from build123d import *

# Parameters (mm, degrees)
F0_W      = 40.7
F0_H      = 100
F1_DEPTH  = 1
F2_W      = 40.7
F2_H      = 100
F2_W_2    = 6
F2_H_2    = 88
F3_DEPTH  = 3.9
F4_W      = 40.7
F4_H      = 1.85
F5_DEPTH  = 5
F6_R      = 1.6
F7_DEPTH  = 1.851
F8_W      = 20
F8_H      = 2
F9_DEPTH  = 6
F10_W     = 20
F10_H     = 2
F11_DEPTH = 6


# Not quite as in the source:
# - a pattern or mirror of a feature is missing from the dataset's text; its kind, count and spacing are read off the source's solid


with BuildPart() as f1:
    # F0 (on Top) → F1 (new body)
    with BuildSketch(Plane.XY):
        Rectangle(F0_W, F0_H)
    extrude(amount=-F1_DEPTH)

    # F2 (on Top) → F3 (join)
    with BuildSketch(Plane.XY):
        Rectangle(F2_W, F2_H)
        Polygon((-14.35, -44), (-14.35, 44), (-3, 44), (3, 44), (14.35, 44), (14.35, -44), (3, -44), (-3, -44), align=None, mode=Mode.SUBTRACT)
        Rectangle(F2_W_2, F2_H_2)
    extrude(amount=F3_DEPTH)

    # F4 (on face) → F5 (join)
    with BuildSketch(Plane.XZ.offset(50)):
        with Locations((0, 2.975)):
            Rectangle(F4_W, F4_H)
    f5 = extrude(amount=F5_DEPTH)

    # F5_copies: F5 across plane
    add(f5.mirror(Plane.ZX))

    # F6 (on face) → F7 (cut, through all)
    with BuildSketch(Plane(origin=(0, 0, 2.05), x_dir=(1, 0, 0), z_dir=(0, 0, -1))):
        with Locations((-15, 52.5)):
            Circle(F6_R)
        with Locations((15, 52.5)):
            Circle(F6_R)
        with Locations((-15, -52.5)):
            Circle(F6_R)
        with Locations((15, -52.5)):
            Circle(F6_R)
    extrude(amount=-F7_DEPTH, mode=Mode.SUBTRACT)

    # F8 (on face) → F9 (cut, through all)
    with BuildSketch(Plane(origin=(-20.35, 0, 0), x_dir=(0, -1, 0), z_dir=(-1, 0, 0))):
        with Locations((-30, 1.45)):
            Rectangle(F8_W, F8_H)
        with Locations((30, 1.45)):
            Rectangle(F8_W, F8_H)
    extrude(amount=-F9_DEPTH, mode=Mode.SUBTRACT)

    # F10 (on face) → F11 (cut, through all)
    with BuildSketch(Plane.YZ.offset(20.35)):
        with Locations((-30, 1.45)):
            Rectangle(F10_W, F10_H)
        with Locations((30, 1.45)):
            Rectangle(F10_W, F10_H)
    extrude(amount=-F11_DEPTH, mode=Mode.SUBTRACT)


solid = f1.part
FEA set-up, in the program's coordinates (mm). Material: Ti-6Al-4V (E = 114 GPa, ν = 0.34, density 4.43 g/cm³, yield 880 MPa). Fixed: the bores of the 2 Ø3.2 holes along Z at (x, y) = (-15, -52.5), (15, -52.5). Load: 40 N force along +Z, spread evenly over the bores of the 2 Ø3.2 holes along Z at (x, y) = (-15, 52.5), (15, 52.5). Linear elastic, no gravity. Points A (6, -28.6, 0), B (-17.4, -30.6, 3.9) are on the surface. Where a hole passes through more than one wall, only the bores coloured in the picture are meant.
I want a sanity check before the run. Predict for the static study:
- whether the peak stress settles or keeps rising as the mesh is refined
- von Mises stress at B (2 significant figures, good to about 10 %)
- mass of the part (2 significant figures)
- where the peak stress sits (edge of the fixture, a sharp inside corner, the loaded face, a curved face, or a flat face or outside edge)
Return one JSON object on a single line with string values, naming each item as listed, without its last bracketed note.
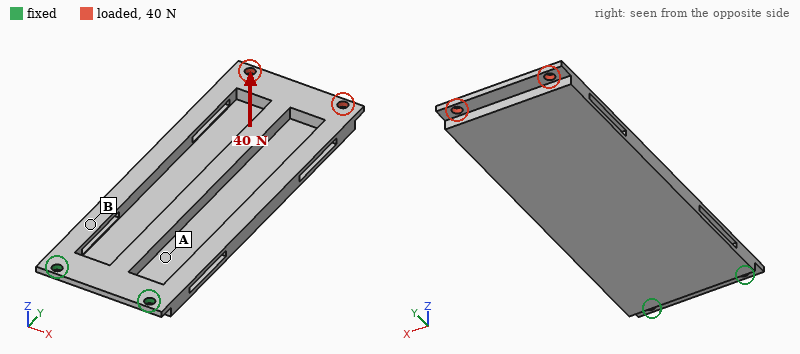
{"whether the peak stress settles or keeps rising as the mesh is refined": "keeps rising", "von Mises stress at B": "43 MPa", "mass of the part": "53 g", "where the peak stress sits": "edge of the fixture"}
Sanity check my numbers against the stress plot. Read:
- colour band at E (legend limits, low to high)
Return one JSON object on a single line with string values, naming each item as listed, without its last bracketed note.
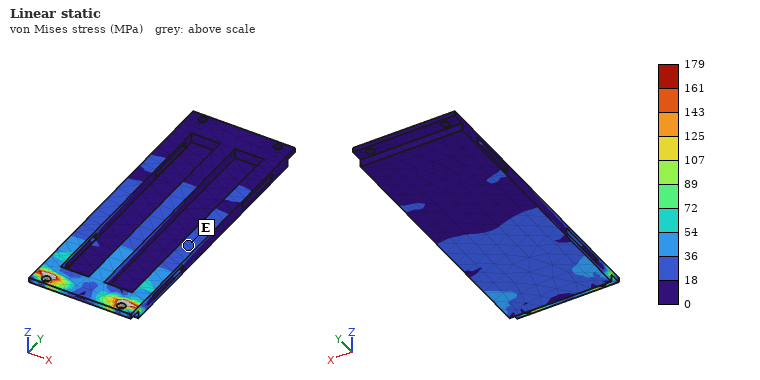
{"colour band at E": "18 to 36 MPa"}
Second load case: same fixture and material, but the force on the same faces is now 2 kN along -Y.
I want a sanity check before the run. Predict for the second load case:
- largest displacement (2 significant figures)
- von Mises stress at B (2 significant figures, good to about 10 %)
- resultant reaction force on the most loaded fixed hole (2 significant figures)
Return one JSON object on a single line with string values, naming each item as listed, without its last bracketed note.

{"largest displacement": "0.80 mm", "von Mises stress at B": "80 MPa", "resultant reaction force on the most loaded fixed hole": "1.0 kN"}
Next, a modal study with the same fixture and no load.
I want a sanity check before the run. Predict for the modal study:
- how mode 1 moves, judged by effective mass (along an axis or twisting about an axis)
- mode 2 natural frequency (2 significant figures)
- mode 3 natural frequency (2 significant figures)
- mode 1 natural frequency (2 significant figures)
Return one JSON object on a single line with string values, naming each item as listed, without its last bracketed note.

{"how mode 1 moves, judged by effective mass": "along Z", "mode 2 natural frequency": "940 Hz", "mode 3 natural frequency": "1600 Hz", "mode 1 natural frequency": "220 Hz"}
